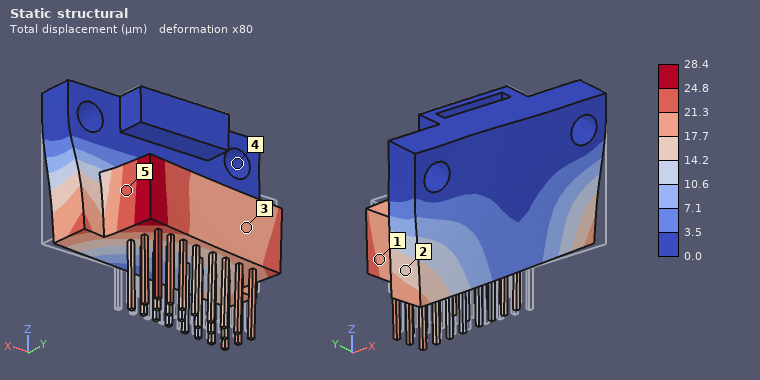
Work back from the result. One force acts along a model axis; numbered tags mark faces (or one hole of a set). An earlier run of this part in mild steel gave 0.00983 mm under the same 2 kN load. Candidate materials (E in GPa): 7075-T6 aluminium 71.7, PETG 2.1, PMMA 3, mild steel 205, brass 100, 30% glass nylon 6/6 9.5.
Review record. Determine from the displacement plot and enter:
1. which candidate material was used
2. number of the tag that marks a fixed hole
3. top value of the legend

7075-T6 aluminium
4
28.4 µm
